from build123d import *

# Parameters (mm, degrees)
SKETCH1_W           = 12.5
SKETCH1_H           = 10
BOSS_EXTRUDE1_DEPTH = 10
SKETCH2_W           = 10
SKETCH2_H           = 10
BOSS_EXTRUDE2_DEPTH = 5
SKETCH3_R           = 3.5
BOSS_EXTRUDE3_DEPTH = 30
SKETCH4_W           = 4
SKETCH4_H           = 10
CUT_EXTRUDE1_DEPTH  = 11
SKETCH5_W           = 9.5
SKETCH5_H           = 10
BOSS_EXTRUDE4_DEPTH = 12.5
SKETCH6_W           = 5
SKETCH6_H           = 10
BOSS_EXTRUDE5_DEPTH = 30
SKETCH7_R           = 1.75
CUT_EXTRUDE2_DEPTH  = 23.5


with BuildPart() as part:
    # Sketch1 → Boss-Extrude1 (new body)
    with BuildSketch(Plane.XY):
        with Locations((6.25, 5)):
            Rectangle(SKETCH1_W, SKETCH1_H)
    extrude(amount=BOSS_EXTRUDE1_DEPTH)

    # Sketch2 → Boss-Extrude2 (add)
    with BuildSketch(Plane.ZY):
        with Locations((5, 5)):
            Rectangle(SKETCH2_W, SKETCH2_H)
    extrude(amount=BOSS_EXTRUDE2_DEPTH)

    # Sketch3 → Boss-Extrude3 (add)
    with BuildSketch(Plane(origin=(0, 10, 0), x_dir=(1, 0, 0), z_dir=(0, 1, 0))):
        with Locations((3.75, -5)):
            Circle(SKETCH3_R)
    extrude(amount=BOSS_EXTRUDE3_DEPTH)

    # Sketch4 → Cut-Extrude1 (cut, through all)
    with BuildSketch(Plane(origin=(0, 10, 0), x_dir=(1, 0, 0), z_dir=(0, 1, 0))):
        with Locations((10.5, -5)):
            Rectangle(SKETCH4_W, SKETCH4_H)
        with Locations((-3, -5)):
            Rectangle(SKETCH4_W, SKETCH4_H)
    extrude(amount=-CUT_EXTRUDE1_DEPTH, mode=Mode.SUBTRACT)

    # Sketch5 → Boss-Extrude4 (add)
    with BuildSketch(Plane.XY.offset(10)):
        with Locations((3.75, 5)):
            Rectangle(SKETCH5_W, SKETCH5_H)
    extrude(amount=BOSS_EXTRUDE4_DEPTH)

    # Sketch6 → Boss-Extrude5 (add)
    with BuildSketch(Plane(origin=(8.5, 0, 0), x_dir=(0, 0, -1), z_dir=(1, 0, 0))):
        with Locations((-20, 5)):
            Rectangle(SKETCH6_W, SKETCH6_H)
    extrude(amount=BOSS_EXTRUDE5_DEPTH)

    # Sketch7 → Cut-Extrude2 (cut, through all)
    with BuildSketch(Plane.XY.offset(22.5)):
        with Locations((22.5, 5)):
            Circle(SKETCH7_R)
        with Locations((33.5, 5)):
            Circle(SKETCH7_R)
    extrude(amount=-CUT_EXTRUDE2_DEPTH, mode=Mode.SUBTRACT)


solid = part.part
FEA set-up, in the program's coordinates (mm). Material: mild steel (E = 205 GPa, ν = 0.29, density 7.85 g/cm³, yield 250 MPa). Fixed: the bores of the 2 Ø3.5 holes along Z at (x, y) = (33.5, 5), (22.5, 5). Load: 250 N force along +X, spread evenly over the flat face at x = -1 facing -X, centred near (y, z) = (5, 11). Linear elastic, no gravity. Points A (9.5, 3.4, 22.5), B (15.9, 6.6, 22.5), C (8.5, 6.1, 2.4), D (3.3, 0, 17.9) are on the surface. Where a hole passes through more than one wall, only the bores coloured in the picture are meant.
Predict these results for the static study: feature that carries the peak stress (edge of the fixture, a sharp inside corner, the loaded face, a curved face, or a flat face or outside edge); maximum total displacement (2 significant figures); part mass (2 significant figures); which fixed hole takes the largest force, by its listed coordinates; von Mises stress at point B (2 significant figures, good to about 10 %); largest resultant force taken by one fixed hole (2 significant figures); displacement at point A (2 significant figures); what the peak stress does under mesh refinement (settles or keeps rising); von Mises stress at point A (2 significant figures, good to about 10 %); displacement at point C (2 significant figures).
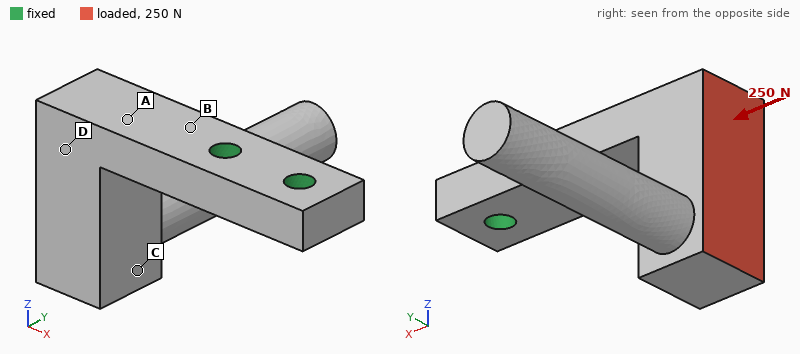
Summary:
edge of the fixture
42 µm
37 g
(22.5, 5)
47 MPa
230 N
8.4 µm
keeps rising
42 MPa
31 µm
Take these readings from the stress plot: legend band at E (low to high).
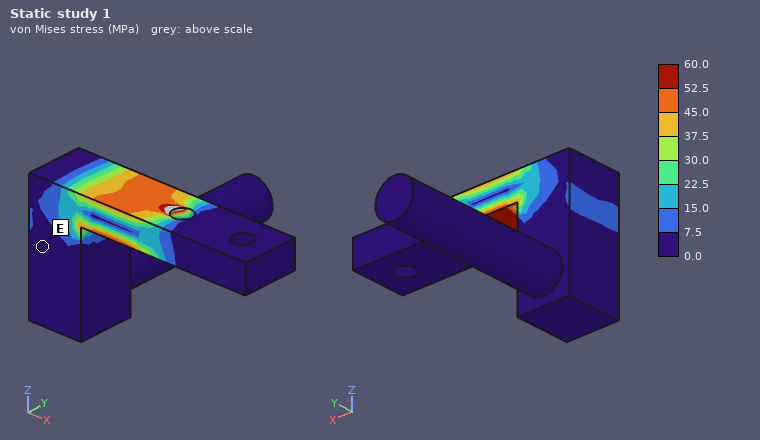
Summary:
0.0 to 7.5 MPa
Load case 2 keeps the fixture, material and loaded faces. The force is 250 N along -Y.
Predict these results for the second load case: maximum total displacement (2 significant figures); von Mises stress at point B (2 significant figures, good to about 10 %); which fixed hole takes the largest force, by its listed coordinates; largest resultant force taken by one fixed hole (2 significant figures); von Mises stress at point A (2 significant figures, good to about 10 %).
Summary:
70 µm
45 MPa
(22.5, 5)
470 N
27 MPa
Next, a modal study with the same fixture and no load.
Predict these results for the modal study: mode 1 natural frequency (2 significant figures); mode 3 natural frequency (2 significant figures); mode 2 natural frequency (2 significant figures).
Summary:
1800 Hz
3900 Hz
2100 Hz
